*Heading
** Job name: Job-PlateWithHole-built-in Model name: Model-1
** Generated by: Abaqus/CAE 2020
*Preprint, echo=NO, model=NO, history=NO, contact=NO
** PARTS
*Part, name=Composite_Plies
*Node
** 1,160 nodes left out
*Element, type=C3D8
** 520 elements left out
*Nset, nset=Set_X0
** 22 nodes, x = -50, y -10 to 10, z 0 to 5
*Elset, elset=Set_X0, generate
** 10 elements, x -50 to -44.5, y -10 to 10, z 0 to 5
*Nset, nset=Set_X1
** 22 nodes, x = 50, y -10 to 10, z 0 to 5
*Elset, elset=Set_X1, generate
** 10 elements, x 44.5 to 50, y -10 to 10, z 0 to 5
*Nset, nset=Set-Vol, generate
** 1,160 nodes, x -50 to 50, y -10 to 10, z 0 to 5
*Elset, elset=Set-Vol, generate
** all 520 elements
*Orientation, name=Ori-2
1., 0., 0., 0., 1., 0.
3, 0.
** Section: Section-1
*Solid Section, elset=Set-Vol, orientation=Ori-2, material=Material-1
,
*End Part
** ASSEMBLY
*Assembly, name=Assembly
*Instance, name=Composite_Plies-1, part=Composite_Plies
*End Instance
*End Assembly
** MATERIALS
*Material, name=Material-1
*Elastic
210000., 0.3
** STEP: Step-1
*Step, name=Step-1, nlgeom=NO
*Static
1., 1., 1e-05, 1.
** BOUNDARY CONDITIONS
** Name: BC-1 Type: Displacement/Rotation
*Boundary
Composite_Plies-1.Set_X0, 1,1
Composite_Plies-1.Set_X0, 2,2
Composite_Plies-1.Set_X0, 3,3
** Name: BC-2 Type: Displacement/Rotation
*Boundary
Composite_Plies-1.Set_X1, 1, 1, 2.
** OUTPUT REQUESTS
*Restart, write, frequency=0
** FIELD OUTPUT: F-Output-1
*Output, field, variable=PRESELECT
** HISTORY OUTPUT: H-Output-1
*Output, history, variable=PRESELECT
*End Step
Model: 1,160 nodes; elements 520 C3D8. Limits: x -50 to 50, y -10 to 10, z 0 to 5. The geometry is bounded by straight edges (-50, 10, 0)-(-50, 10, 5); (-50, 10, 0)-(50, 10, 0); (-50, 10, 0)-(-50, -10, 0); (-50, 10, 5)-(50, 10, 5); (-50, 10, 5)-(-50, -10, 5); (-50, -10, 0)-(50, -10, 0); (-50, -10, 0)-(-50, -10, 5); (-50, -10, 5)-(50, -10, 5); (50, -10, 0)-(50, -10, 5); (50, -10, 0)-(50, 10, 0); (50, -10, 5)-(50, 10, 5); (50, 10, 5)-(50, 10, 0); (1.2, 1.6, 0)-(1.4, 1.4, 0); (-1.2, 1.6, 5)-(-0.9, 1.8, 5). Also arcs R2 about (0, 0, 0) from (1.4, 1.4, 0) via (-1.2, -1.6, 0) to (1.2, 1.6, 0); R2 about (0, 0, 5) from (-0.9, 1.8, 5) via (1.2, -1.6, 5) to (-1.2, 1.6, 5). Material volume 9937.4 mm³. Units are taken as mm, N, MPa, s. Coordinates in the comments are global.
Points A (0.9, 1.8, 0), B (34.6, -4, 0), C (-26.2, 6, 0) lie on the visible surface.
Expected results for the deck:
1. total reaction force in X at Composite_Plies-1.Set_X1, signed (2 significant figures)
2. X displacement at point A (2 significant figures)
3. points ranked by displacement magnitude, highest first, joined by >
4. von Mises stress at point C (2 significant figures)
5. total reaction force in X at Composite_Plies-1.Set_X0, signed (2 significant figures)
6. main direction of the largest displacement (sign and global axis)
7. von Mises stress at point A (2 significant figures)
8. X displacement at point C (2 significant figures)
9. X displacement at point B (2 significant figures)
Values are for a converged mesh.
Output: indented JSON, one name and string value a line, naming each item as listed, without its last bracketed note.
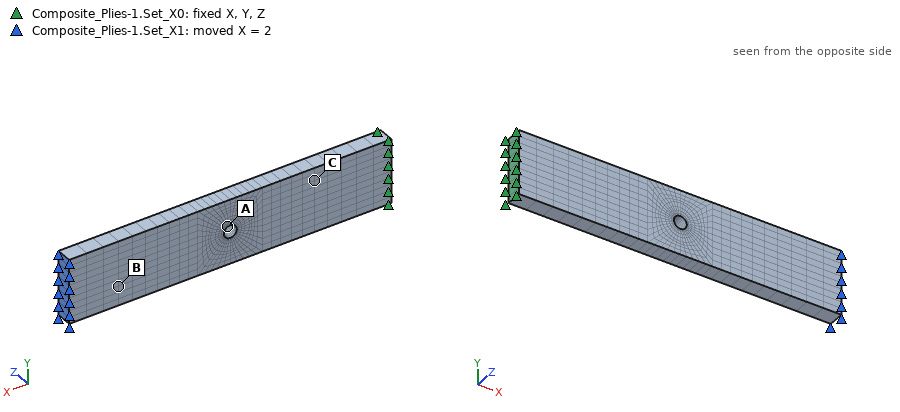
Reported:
{
  "total reaction force in X at Composite_Plies-1.Set_X1, signed": "4.1e+05 N",
  "X displacement at point A": "1.0 mm",
  "points ranked by displacement magnitude, highest first, joined by >": "B > A > C",
  "von Mises stress at point C": "4100 MPa",
  "total reaction force in X at Composite_Plies-1.Set_X0, signed": "-4.1e+05 N",
  "main direction of the largest displacement": "+X",
  "von Mises stress at point A": "8700 MPa",
  "X displacement at point C": "0.46 mm",
  "X displacement at point B": "1.7 mm"
}
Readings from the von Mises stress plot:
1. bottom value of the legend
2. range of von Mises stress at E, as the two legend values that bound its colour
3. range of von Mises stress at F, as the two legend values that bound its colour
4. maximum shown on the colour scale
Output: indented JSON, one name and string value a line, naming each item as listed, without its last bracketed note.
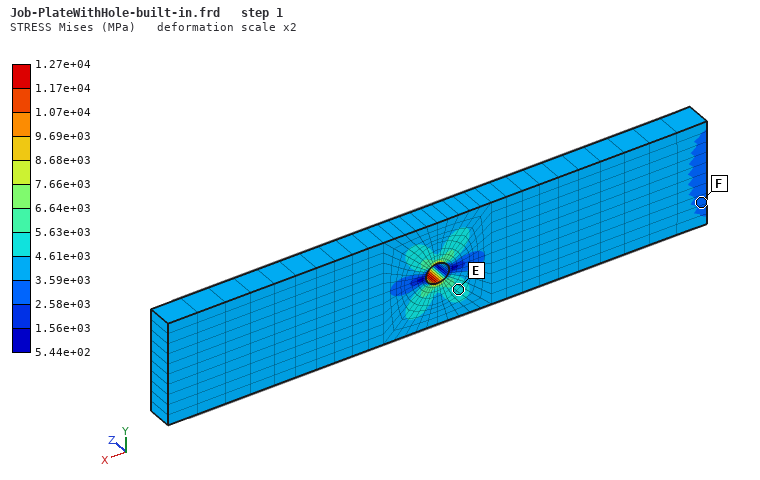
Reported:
{
  "bottom value of the legend": "5.44e+02 MPa",
  "range of von Mises stress at E, as the two legend values that bound its colour": "4.61e+03 to 5.63e+03 MPa",
  "range of von Mises stress at F, as the two legend values that bound its colour": "2.58e+03 to 3.59e+03 MPa",
  "maximum shown on the colour scale": "1.27e+04 MPa"
}
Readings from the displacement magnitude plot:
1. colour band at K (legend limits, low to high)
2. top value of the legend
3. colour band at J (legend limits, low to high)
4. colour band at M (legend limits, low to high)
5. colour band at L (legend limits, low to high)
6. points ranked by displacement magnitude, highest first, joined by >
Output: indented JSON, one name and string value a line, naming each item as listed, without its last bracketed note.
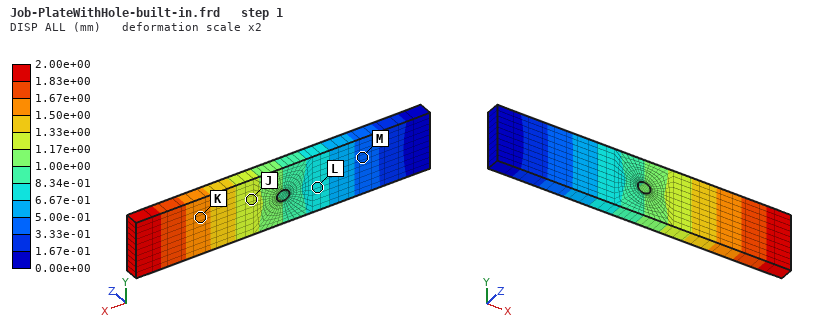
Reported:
{
  "colour band at K": "1.50e+00 to 1.67e+00 mm",
  "top value of the legend": "2.00e+00 mm",
  "colour band at J": "1.17e+00 to 1.33e+00 mm",
  "colour band at M": "3.33e-01 to 5.00e-01 mm",
  "colour band at L": "6.67e-01 to 8.34e-01 mm",
  "points ranked by displacement magnitude, highest first, joined by >": "K > J > L > M"
}
